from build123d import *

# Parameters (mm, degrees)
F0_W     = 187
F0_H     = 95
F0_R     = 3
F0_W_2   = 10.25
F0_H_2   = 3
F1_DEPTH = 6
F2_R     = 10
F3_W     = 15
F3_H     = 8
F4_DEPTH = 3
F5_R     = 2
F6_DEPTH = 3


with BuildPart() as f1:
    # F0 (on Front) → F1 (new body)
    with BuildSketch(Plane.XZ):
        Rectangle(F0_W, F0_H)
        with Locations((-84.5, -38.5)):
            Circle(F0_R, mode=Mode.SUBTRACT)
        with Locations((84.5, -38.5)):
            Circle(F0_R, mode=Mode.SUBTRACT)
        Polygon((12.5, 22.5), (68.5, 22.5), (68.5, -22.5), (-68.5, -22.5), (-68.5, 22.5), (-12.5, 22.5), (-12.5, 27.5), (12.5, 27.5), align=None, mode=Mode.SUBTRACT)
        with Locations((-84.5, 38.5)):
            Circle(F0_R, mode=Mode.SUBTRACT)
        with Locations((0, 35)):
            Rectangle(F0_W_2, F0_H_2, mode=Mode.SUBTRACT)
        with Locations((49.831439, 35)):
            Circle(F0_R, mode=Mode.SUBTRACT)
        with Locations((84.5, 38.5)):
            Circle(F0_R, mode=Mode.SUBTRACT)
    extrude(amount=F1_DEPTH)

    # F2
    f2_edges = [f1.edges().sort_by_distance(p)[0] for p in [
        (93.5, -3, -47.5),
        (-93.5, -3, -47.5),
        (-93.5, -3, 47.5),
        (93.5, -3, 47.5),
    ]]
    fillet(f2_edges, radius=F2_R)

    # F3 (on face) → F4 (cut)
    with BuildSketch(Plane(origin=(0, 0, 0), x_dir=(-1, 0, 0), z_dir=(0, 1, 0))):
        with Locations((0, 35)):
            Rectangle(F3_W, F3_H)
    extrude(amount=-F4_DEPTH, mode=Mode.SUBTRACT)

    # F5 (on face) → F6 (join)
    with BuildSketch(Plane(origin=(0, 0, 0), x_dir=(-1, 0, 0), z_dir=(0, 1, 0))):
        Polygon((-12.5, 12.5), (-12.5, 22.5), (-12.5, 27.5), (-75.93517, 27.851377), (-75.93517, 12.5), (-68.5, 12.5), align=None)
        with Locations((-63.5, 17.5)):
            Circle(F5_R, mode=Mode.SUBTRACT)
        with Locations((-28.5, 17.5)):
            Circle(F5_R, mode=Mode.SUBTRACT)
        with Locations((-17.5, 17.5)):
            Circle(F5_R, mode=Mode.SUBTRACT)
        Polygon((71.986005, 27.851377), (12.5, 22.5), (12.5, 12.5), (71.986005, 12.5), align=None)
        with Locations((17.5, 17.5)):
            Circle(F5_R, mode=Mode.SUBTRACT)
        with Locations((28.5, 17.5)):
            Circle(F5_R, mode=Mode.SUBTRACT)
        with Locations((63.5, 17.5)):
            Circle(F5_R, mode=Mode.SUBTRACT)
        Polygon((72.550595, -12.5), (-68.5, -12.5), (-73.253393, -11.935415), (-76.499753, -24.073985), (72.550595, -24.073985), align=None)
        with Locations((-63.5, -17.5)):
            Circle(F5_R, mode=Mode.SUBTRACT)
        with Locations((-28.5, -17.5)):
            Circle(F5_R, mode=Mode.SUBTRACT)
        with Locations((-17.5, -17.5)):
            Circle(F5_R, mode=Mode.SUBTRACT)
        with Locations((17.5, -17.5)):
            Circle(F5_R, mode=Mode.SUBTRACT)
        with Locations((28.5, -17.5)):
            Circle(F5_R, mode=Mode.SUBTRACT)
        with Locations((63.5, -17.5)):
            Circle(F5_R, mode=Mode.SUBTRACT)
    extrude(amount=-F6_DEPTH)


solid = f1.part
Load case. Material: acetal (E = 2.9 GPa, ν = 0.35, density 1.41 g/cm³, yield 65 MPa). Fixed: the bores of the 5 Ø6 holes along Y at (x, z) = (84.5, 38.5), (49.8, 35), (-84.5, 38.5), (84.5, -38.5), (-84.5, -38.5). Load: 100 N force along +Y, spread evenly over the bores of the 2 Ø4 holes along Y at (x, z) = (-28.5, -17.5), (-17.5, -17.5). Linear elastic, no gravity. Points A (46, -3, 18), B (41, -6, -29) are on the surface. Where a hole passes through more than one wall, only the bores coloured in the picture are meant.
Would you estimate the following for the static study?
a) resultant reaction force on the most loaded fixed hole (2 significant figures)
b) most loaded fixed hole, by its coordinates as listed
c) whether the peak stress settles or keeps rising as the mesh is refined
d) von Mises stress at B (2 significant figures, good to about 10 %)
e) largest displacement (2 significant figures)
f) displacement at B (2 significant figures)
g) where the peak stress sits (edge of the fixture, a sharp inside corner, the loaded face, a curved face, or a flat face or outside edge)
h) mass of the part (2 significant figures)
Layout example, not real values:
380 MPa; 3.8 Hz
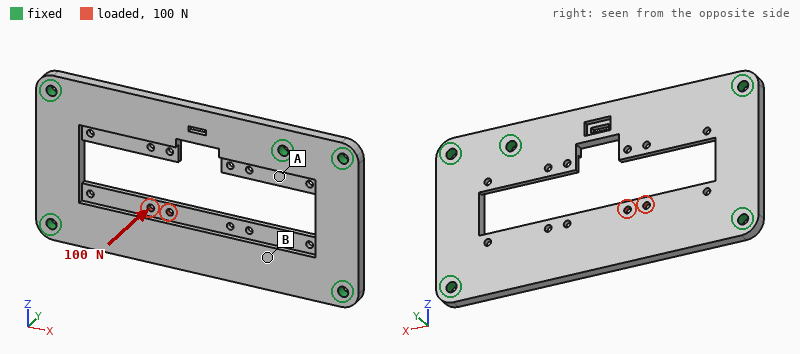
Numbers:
63 N; (-84.5, -38.5); keeps rising; 4.3 MPa; 2.2 mm; 0.68 mm; edge of the fixture; 100 g
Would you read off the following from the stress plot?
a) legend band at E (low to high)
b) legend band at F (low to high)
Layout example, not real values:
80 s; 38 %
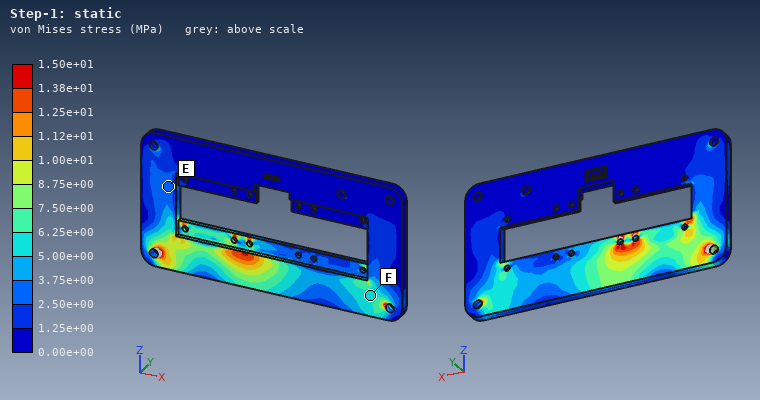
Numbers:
2.50e+00 to 3.75e+00 MPa; 5.00e+00 to 6.25e+00 MPa
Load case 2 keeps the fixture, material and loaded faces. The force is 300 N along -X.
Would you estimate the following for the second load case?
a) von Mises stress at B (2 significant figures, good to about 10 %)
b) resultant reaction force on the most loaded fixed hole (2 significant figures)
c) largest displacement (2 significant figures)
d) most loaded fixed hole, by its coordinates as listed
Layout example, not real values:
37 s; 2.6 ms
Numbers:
0.85 MPa; 170 N; 75 µm; (-84.5, -38.5)
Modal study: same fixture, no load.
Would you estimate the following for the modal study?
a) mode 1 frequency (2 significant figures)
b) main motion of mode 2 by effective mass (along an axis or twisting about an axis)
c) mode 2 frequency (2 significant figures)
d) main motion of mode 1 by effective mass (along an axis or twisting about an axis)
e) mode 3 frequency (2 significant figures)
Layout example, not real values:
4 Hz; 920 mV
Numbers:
300 Hz; along Y; 490 Hz; along Y; 810 Hz
